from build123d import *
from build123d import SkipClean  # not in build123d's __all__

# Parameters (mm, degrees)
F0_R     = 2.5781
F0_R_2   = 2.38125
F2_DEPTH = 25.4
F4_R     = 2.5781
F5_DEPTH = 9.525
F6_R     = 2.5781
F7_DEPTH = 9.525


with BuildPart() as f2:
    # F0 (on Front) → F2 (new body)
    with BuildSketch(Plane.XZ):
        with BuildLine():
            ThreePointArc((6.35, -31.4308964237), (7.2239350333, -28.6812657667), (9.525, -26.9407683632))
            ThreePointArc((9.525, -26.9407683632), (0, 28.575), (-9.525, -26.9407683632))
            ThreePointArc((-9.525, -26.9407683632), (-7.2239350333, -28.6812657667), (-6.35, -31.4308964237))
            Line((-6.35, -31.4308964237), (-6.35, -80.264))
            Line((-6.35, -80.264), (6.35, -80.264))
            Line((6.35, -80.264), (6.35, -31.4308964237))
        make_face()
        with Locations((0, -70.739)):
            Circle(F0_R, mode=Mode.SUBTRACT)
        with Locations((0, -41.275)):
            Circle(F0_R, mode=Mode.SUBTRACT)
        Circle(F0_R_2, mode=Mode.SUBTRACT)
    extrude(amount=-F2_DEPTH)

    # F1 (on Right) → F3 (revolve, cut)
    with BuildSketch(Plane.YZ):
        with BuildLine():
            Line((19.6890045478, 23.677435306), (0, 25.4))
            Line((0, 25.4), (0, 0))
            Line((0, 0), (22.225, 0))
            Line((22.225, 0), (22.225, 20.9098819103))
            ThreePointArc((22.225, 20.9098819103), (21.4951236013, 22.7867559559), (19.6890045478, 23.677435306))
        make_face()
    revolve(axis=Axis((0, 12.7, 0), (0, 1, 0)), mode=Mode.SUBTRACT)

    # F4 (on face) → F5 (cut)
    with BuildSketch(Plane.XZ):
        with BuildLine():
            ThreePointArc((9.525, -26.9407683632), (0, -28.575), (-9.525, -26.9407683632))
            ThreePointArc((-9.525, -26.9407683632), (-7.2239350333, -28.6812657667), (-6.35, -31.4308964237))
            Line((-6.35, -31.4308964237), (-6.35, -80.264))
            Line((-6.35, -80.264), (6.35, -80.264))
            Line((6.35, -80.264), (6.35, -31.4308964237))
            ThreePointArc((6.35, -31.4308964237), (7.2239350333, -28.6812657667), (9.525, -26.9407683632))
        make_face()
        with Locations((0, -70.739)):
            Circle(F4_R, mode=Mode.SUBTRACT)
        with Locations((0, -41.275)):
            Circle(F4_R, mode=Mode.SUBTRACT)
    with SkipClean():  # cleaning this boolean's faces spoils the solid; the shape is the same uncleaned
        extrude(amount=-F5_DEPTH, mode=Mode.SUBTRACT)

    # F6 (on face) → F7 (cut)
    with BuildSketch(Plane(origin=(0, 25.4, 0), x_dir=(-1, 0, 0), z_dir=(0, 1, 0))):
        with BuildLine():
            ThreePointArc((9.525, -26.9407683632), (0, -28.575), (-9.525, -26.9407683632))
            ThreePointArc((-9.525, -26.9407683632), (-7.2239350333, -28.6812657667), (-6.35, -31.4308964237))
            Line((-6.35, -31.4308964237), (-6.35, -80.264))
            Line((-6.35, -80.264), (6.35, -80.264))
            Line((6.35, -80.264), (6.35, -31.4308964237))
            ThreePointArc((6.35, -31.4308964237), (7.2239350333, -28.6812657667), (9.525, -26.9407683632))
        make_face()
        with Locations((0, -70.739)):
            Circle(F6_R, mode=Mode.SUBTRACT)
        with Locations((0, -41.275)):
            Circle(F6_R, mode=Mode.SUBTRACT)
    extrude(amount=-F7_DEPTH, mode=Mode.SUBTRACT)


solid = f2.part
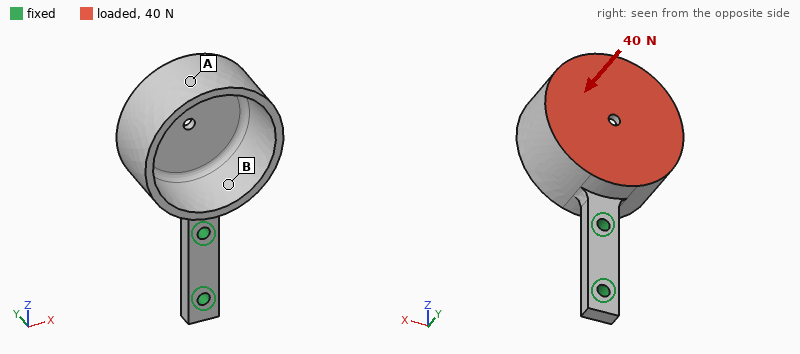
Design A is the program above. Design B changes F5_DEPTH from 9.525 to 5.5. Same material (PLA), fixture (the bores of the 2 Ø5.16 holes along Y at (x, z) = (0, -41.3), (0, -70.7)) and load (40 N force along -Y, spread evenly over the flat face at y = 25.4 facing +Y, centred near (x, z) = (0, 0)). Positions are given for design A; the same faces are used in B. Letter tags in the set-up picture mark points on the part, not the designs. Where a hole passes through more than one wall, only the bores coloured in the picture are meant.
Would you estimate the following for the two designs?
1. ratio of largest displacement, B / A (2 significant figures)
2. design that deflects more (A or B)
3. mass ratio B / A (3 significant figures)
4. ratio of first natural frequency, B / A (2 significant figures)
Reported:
0.38
A
1.09
1.6
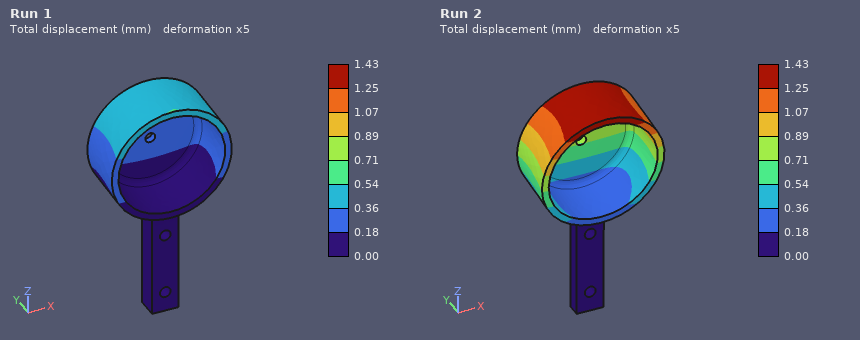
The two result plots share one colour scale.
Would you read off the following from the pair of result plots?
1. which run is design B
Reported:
Run 1
